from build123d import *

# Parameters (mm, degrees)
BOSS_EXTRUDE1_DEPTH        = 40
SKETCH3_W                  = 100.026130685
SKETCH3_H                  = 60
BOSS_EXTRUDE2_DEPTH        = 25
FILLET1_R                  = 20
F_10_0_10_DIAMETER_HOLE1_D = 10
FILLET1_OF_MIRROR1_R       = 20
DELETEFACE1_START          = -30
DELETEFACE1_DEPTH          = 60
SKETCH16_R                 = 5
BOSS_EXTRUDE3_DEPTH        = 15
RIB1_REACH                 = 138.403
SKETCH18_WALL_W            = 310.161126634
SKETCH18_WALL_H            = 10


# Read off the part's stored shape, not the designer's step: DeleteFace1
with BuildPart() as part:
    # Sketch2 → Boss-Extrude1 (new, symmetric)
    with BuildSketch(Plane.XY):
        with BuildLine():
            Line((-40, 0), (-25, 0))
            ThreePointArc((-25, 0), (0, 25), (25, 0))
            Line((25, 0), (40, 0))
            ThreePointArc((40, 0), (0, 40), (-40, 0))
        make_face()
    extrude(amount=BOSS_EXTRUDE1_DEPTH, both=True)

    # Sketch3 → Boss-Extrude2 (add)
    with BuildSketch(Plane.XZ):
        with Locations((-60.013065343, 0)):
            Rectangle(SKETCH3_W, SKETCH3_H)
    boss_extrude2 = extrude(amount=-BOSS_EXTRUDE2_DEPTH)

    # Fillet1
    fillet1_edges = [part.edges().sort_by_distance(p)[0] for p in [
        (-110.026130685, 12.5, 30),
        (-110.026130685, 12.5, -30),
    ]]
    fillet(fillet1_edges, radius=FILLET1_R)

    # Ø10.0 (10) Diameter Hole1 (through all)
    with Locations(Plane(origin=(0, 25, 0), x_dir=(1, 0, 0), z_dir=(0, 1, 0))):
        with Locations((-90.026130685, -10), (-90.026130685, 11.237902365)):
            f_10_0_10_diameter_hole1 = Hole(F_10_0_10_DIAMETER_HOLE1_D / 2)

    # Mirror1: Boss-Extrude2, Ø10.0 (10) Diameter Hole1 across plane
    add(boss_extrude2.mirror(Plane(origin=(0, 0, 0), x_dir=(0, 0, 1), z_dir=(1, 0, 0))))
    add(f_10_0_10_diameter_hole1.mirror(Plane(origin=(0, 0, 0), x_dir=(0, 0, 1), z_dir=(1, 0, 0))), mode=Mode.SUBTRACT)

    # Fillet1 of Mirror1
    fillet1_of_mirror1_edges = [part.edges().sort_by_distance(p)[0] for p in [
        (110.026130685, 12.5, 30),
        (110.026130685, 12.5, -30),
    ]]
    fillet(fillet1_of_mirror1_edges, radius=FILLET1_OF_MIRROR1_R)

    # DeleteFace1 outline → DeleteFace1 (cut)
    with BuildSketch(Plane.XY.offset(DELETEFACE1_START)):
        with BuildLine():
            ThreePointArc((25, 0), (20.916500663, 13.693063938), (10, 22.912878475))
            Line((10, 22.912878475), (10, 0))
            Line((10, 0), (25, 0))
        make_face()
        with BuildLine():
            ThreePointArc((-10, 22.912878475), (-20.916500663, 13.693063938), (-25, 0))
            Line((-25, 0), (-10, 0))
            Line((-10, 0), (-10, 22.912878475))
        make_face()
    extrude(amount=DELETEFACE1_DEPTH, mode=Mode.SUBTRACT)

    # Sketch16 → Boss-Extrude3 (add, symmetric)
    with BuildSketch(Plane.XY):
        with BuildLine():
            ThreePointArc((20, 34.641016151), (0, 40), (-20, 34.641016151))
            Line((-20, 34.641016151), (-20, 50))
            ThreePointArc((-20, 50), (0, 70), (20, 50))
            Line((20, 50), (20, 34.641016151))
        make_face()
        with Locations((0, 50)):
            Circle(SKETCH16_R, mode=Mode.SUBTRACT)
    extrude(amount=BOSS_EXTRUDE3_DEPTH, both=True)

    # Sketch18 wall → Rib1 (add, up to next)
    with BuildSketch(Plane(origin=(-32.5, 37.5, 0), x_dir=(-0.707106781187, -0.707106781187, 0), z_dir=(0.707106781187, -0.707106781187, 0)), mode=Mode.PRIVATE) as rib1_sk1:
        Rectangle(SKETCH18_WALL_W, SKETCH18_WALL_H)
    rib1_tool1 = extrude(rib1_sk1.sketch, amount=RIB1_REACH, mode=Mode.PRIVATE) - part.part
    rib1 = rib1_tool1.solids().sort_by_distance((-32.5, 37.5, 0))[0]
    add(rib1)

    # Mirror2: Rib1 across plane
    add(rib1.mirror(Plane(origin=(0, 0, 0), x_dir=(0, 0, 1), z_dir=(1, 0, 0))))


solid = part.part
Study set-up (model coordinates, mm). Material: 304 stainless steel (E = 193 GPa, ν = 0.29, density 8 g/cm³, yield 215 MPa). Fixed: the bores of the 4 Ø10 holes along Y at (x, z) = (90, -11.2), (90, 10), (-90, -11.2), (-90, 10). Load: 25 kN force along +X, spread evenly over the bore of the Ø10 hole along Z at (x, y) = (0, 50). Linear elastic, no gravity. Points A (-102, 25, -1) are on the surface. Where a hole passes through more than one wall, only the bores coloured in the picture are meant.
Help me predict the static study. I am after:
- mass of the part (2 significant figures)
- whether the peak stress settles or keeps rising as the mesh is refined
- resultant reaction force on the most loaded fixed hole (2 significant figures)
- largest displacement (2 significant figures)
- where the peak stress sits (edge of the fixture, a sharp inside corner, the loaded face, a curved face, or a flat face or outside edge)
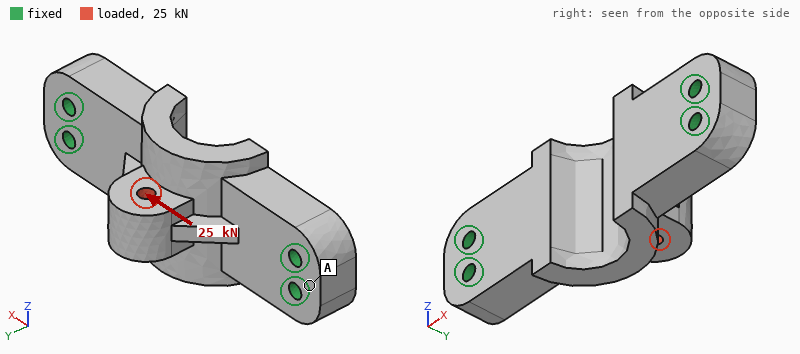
2.9 kg
keeps rising
7.5 kN
32 µm
edge of the fixture
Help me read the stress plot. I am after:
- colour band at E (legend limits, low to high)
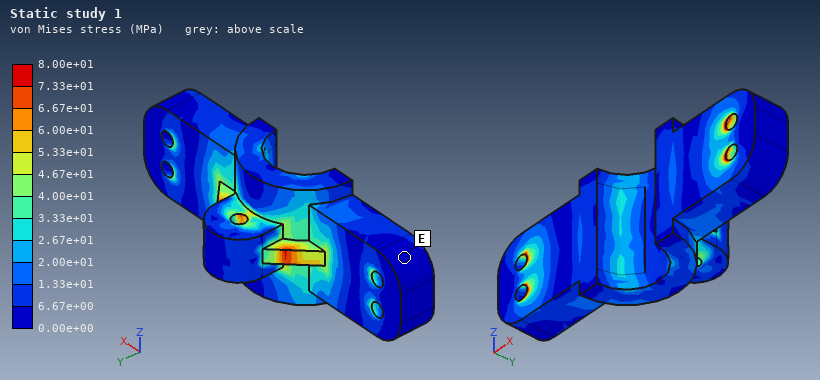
0.00e+00 to 6.67e+00 MPa
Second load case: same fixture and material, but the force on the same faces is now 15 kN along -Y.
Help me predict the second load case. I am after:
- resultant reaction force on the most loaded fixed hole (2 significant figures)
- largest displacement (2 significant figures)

7.2 kN
26 µm
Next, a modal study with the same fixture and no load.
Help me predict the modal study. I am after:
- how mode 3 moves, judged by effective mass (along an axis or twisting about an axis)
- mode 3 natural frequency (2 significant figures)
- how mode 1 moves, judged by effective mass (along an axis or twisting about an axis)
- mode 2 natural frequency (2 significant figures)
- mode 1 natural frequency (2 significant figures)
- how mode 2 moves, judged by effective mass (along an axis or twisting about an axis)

along Z
5800 Hz
along Z
3400 Hz
3000 Hz
along Y
